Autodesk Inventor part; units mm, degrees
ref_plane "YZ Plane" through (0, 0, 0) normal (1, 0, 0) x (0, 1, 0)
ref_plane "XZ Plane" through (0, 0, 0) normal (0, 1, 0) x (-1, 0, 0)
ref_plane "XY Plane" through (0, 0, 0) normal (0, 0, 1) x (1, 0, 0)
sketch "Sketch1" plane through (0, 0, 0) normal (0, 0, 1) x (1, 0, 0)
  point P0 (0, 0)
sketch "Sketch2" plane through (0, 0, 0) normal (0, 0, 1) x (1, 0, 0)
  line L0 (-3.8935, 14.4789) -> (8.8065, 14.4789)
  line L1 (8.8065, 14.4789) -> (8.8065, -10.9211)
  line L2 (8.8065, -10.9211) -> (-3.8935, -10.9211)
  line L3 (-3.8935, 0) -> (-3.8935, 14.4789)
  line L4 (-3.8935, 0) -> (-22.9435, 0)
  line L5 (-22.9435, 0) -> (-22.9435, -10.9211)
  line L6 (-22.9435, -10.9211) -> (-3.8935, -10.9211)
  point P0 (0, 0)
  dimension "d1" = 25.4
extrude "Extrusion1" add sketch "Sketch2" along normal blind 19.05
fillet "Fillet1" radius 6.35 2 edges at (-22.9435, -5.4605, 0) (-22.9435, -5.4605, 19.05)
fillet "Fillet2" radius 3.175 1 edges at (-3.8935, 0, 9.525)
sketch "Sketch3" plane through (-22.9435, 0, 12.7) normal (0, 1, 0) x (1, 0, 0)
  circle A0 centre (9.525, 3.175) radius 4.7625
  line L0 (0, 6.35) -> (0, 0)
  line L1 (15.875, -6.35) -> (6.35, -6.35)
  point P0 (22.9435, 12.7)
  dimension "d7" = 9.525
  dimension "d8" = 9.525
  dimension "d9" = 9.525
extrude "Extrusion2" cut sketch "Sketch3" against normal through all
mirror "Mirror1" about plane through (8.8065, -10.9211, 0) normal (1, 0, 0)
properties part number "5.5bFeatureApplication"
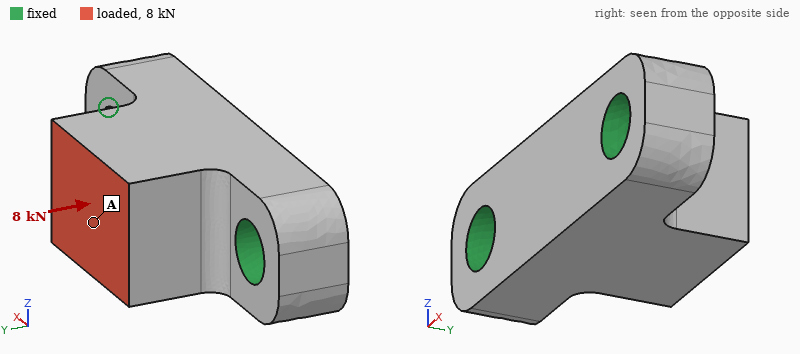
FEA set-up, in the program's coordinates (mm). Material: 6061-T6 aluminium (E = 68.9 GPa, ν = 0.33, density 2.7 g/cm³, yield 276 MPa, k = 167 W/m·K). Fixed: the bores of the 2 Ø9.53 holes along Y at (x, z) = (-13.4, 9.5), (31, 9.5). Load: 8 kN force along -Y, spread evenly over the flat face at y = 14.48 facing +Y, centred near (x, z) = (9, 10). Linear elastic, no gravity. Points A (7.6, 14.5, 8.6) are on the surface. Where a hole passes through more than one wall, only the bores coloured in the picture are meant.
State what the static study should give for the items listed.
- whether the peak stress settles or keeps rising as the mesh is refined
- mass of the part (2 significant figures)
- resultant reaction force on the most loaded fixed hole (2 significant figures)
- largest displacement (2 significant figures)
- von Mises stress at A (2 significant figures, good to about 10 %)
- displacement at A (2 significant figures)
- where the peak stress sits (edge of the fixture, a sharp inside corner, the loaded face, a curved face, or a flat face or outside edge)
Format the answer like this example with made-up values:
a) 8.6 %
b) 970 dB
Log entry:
a) keeps rising
b) 50 g
c) 4.3 kN
d) 14 µm
e) 14 MPa
f) 14 µm
g) edge of the fixture
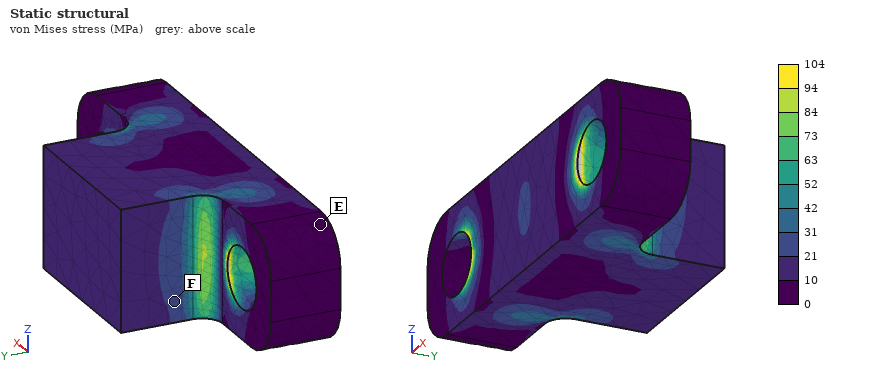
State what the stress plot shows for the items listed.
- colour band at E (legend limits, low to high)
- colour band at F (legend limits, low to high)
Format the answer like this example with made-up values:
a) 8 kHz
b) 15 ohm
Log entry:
a) 0 to 10 MPa
b) 21 to 31 MPa
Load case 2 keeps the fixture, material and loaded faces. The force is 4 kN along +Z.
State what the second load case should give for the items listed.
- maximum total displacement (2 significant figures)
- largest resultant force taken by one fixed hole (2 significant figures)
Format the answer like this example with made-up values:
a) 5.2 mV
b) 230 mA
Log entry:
a) 67 µm
b) 2.0 kN
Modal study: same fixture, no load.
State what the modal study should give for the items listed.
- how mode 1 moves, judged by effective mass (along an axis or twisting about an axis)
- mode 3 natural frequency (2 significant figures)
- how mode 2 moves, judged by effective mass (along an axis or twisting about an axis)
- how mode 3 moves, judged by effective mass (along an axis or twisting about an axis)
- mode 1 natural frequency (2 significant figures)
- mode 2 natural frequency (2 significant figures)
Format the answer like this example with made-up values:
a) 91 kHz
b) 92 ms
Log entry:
a) along Z
b) 27 kHz
c) along Y
d) along X
e) 12 kHz
f) 23 kHz
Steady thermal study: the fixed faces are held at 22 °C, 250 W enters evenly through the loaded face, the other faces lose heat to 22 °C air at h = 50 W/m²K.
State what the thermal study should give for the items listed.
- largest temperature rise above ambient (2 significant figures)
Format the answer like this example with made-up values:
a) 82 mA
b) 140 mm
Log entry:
a) 86 K
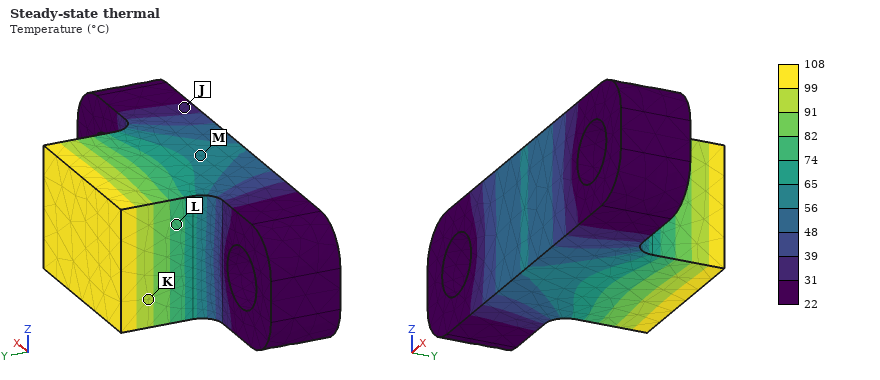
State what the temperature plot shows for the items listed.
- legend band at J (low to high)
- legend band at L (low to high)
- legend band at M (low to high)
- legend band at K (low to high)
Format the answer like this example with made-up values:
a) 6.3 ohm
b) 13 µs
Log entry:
a) 31 to 39 °C
b) 74 to 82 °C
c) 56 to 65 °C
d) 91 to 99 °C
